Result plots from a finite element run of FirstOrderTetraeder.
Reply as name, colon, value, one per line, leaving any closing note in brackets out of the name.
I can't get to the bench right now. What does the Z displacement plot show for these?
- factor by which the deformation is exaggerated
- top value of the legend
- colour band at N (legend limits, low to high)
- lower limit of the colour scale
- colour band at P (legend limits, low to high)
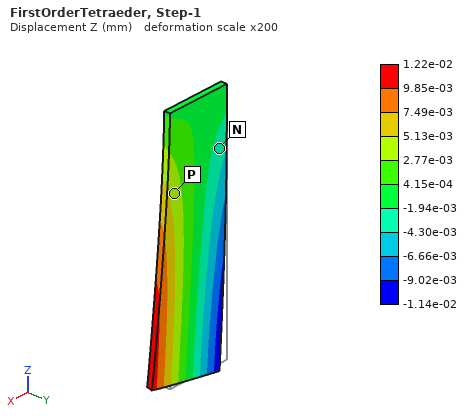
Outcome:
factor by which the deformation is exaggerated: 200
top value of the legend: 1.22e-02 mm
colour band at N: -4.30e-03 to -1.94e-03 mm
lower limit of the colour scale: -1.14e-02 mm
colour band at P: 2.77e-03 to 5.13e-03 mm
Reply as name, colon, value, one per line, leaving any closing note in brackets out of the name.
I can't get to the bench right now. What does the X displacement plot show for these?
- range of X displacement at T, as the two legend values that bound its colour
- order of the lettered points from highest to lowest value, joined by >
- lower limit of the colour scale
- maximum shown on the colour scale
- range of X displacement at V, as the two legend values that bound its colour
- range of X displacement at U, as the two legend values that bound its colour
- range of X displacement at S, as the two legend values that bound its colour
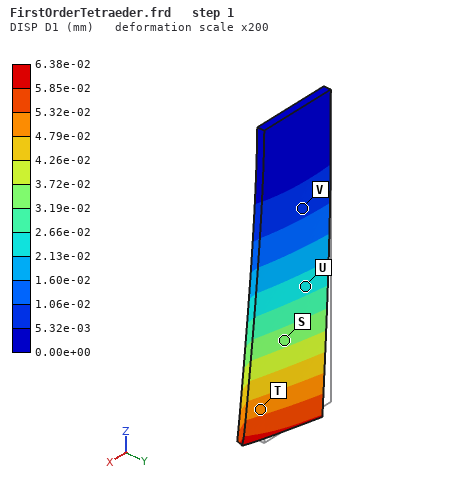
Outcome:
range of X displacement at T, as the two legend values that bound its colour: 4.79e-02 to 5.32e-02 mm
order of the lettered points from highest to lowest value, joined by >: T > S > U > V
lower limit of the colour scale: 0.00e+00 mm
maximum shown on the colour scale: 6.38e-02 mm
range of X displacement at V, as the two legend values that bound its colour: 5.32e-03 to 1.06e-02 mm
range of X displacement at U, as the two legend values that bound its colour: 2.13e-02 to 2.66e-02 mm
range of X displacement at S, as the two legend values that bound its colour: 3.19e-02 to 3.72e-02 mm
